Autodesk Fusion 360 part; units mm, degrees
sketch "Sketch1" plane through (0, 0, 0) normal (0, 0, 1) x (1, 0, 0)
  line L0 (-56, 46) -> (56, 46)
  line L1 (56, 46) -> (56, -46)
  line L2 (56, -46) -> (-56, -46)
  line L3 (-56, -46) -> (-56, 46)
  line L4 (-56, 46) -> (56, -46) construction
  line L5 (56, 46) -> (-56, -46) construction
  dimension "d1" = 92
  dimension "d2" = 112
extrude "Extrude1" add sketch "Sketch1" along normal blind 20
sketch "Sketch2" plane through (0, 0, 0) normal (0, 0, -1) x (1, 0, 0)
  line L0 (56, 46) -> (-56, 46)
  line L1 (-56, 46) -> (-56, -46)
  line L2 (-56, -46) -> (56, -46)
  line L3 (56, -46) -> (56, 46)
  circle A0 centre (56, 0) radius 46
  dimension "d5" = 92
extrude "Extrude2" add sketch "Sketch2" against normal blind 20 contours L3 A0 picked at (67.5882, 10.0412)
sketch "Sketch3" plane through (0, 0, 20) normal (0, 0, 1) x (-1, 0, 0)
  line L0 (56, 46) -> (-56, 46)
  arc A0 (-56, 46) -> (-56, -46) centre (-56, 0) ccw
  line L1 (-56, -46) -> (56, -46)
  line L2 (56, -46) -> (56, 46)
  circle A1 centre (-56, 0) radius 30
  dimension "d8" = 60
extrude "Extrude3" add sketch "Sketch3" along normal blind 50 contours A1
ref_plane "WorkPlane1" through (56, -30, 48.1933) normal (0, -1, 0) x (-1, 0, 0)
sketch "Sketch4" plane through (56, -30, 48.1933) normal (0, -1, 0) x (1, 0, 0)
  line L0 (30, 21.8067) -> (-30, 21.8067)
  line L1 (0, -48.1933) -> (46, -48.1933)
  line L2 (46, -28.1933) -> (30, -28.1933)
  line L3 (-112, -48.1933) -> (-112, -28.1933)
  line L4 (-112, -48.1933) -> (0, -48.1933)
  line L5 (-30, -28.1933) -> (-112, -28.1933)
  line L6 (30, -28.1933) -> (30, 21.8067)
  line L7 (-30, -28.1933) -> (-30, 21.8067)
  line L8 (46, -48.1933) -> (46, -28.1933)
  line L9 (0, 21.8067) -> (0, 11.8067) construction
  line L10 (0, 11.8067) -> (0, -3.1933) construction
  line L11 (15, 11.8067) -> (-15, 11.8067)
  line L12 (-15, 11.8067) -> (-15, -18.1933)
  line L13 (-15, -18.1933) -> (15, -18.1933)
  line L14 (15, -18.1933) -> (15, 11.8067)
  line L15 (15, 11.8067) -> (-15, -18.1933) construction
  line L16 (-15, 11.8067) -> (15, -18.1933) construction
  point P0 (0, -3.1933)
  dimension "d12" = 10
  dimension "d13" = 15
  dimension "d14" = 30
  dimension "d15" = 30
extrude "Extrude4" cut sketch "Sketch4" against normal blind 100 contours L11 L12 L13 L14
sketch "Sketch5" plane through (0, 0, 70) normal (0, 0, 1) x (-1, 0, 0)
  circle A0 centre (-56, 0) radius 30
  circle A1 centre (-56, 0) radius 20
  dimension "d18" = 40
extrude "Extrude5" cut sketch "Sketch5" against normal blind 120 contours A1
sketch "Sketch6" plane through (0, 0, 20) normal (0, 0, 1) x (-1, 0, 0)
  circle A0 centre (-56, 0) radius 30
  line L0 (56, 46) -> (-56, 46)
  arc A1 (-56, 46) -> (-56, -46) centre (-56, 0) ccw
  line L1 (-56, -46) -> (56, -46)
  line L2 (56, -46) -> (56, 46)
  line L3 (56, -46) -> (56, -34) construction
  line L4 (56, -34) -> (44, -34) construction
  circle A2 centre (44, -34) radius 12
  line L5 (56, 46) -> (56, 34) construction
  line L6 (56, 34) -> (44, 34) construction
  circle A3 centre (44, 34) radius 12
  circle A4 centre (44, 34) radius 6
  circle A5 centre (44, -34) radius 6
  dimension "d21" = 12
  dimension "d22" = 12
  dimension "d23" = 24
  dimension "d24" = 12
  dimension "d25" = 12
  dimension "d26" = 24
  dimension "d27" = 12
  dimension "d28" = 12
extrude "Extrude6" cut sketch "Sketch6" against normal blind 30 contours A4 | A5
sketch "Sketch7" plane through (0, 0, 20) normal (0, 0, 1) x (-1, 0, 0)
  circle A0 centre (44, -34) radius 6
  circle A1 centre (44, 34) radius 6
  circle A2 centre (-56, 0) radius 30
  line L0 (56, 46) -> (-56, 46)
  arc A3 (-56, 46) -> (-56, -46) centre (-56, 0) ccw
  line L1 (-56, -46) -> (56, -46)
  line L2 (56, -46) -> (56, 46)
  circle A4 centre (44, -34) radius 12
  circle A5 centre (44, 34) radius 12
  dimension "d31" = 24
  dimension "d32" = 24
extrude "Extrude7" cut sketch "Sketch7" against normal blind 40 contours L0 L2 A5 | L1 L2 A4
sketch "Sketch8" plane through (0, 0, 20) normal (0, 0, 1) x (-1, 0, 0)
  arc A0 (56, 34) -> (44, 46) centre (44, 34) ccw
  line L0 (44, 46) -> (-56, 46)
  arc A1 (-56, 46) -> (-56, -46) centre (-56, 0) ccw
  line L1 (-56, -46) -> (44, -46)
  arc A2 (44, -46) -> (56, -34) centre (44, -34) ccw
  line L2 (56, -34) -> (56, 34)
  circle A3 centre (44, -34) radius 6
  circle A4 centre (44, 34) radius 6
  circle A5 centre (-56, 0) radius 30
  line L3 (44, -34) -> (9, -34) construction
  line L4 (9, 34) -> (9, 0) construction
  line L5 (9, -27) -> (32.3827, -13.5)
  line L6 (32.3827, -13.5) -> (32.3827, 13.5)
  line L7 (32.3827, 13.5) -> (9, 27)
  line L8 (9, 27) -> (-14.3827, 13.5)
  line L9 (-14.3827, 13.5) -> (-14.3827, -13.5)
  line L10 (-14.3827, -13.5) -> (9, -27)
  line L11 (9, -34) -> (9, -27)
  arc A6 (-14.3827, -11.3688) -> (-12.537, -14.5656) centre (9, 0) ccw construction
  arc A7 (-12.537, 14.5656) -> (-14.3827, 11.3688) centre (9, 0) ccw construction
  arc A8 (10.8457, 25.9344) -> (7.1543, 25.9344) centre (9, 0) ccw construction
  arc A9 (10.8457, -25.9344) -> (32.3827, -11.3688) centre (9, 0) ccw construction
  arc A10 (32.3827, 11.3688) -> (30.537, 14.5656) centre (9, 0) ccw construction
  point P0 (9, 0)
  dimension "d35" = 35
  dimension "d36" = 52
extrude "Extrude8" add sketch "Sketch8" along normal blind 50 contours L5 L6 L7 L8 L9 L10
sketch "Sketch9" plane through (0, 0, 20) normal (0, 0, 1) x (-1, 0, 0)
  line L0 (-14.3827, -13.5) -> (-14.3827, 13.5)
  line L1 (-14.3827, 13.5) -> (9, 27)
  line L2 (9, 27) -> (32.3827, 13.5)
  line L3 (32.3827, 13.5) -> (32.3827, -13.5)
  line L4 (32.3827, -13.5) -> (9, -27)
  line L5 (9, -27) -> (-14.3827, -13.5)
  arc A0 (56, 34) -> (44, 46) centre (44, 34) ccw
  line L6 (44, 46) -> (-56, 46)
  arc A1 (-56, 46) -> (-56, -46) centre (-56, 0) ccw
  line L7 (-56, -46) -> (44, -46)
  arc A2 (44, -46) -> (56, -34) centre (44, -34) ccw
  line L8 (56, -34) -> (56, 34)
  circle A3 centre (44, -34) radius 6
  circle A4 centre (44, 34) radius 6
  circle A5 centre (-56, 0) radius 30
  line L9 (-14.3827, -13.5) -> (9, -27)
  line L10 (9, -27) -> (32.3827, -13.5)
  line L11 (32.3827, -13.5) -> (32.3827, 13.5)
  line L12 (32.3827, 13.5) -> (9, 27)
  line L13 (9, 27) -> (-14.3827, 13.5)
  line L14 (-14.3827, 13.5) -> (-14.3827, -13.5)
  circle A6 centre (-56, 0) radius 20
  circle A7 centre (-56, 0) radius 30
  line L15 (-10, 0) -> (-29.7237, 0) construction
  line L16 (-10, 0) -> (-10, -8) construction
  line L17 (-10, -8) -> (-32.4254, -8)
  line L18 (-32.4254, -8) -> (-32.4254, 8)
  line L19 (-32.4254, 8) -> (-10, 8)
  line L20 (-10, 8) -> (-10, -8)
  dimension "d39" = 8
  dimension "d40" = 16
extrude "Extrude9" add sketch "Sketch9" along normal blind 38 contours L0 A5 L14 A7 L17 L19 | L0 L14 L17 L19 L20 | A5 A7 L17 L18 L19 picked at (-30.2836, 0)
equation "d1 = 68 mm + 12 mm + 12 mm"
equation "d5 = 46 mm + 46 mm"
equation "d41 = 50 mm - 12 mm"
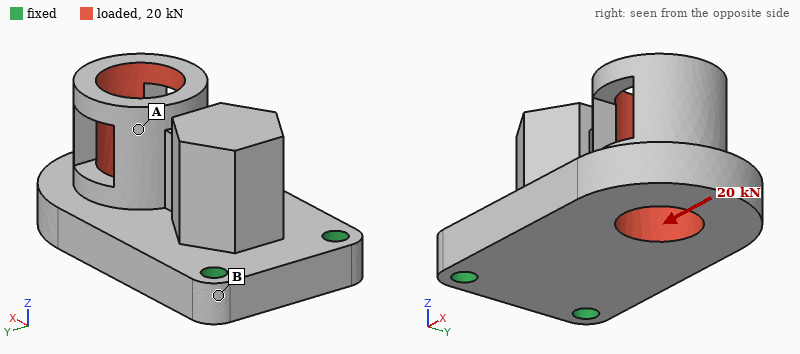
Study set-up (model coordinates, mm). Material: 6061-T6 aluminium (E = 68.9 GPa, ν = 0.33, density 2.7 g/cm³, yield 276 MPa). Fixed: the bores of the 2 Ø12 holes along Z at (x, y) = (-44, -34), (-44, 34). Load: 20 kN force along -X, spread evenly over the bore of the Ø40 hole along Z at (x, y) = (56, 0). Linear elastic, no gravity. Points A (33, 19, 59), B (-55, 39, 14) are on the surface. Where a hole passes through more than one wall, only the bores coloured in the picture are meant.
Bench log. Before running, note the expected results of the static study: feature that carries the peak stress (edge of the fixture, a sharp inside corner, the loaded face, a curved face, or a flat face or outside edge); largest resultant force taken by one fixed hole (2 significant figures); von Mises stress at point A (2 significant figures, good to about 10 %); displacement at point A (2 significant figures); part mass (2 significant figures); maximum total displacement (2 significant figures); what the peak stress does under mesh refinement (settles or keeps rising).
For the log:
edge of the fixture
10 kN
32 MPa
0.29 mm
1.1 kg
0.53 mm
keeps rising
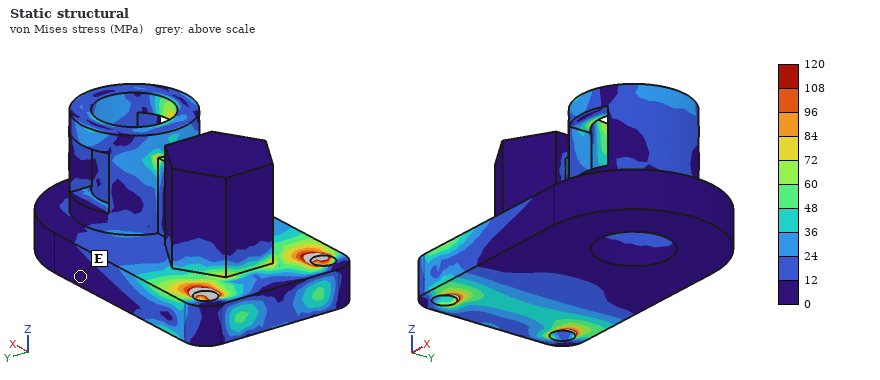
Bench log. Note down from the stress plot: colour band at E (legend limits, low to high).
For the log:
0 to 12 MPa
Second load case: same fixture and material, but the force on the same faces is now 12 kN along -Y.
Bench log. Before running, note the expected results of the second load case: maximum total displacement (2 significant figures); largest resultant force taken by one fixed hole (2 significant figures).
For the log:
0.18 mm
18 kN
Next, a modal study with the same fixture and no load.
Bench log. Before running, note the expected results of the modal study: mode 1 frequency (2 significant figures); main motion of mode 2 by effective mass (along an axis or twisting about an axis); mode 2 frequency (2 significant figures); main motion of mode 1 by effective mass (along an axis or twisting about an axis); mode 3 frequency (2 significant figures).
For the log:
800 Hz
along Y
2400 Hz
along Z
3000 Hz
